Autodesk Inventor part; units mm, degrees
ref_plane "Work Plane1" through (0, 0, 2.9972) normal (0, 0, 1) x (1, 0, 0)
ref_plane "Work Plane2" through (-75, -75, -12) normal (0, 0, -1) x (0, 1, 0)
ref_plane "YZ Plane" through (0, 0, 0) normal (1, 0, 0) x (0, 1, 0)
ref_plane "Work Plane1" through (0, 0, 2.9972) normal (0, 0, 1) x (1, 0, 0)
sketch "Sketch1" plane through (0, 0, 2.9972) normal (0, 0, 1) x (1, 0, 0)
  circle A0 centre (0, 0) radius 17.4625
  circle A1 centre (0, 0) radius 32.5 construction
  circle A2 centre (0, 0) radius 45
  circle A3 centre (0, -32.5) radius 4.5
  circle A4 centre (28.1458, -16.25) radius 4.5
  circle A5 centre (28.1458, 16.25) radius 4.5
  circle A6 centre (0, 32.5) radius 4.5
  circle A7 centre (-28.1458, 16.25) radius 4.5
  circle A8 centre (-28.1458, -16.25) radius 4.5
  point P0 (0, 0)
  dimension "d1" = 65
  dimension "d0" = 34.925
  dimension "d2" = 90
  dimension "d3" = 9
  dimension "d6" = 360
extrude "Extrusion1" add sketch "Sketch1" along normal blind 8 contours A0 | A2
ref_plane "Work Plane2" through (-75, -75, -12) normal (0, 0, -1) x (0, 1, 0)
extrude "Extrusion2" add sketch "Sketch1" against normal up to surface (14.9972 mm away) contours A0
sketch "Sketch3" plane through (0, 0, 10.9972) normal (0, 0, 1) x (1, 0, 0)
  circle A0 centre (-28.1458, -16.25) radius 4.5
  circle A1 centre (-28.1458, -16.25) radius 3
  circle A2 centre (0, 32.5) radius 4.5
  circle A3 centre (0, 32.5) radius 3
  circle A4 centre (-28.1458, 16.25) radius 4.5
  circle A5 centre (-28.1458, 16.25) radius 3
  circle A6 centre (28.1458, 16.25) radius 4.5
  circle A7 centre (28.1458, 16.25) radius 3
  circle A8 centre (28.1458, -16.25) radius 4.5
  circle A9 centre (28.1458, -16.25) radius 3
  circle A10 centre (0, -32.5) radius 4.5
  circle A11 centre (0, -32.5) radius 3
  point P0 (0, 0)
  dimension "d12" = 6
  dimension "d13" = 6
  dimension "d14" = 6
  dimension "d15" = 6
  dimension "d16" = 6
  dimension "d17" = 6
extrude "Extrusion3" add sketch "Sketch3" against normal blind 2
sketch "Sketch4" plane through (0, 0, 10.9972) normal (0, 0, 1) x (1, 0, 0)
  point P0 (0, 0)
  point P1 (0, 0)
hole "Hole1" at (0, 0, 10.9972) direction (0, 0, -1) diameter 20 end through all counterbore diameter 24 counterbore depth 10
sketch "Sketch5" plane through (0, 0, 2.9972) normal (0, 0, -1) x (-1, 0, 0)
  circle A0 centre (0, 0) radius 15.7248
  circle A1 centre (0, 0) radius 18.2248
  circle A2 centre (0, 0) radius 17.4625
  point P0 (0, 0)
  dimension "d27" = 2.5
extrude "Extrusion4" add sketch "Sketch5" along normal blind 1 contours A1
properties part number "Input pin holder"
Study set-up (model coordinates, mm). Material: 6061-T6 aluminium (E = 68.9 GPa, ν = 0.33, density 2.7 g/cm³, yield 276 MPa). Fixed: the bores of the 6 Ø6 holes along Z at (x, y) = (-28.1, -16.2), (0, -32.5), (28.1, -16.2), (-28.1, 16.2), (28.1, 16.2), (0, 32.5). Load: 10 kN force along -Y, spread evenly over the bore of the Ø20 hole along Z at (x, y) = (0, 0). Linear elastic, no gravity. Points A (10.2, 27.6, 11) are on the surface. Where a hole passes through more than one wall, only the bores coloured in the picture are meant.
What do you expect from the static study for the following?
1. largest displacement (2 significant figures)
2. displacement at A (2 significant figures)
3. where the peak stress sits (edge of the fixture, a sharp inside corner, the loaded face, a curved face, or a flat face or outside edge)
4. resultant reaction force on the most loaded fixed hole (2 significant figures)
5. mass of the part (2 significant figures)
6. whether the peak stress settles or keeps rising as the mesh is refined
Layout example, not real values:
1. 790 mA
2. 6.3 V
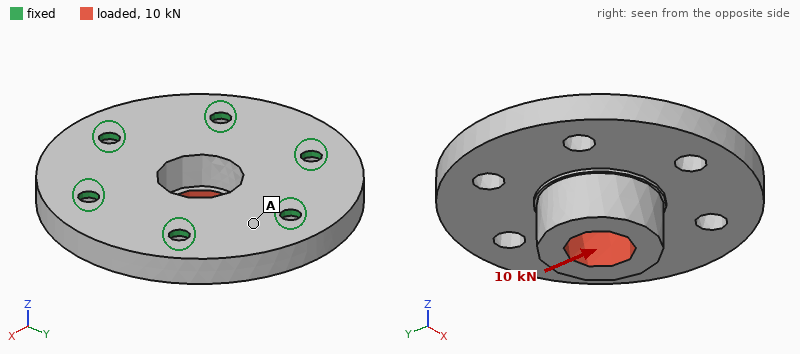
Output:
1. 36 µm
2. 8.8 µm
3. edge of the fixture
4. 3.0 kN
5. 150 g
6. keeps rising
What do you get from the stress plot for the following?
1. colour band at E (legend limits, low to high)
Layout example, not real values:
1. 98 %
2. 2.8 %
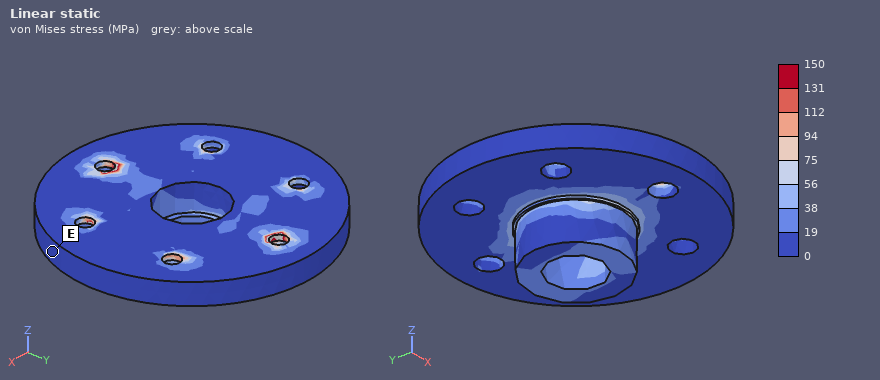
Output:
1. 0 to 19 MPa
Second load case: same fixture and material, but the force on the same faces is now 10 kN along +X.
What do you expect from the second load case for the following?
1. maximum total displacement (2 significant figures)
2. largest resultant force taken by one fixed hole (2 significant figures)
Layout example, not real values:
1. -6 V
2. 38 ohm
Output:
1. 36 µm
2. 2.7 kN
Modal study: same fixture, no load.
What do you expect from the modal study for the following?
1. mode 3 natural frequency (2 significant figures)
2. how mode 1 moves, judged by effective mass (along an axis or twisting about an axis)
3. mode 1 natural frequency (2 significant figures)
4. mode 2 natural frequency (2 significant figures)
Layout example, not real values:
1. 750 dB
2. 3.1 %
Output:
1. 14 kHz
2. along Z
3. 12 kHz
4. 14 kHz
